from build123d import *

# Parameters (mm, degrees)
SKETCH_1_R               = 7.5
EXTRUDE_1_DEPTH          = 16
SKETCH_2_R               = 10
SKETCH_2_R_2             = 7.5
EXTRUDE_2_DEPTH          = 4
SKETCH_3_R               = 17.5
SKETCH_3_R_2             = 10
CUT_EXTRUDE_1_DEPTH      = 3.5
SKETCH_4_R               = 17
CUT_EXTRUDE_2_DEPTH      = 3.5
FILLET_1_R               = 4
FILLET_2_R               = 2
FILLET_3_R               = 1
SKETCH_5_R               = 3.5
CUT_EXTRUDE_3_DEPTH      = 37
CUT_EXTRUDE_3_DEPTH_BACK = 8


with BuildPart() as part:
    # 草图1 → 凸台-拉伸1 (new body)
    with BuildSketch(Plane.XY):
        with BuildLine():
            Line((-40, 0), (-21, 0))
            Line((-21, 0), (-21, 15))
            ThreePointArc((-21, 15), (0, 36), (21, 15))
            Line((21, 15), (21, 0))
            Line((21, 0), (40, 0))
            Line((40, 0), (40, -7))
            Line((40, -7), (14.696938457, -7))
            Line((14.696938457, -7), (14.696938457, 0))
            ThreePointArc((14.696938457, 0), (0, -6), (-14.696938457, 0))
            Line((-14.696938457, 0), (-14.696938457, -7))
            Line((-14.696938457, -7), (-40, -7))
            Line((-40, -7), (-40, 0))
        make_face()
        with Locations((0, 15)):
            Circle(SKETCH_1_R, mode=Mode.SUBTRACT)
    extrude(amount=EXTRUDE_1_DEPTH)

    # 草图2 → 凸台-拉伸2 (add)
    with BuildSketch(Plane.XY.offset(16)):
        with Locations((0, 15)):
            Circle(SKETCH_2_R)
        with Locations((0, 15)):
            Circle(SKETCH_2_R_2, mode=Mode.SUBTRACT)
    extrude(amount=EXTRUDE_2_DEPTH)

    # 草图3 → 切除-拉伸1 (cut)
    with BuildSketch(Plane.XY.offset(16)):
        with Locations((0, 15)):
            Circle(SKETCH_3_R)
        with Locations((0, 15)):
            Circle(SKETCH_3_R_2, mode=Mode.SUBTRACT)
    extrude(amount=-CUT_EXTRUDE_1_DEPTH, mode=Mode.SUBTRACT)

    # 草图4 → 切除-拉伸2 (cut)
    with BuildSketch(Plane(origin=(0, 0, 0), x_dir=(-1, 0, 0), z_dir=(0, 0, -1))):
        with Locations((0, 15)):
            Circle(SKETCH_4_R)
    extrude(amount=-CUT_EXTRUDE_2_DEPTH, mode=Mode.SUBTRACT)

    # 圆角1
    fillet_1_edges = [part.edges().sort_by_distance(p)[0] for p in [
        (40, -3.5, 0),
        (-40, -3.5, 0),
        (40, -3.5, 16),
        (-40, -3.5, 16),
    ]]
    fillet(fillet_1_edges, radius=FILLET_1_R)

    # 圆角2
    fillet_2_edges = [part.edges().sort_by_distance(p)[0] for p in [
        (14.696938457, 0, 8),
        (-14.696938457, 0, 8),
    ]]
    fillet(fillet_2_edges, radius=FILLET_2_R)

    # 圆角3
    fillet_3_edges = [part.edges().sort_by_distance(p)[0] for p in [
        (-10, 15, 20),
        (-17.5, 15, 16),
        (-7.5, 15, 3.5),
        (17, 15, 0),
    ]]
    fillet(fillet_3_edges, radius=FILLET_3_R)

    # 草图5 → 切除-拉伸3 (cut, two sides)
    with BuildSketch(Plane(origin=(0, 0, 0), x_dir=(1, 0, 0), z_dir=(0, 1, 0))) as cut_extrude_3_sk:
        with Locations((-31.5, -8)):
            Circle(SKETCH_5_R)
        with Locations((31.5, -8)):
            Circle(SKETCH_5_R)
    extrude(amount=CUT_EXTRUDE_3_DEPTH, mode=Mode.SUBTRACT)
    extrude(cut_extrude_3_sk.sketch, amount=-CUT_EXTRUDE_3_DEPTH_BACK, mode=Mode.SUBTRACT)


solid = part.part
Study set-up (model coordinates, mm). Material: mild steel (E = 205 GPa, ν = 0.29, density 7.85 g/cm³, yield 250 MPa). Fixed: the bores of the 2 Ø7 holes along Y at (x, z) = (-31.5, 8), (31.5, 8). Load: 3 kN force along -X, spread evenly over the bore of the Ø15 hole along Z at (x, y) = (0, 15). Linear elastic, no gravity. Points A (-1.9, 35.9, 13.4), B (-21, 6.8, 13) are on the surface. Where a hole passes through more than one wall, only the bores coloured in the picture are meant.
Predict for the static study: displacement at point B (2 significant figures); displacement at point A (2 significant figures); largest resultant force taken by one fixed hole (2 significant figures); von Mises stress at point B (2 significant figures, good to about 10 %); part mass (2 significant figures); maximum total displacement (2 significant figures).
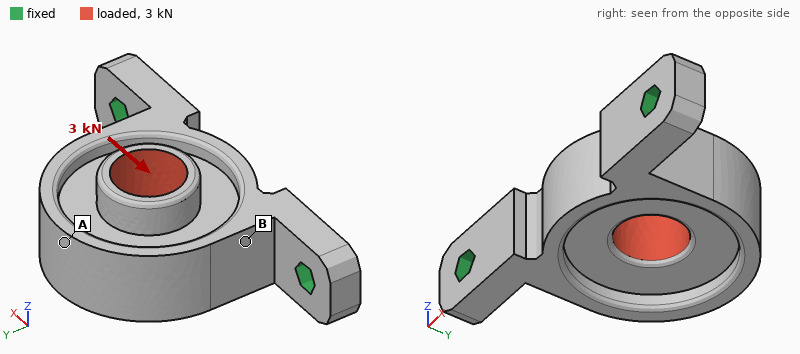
4.2 µm
9.8 µm
1.9 kN
16 MPa
170 g
11 µm
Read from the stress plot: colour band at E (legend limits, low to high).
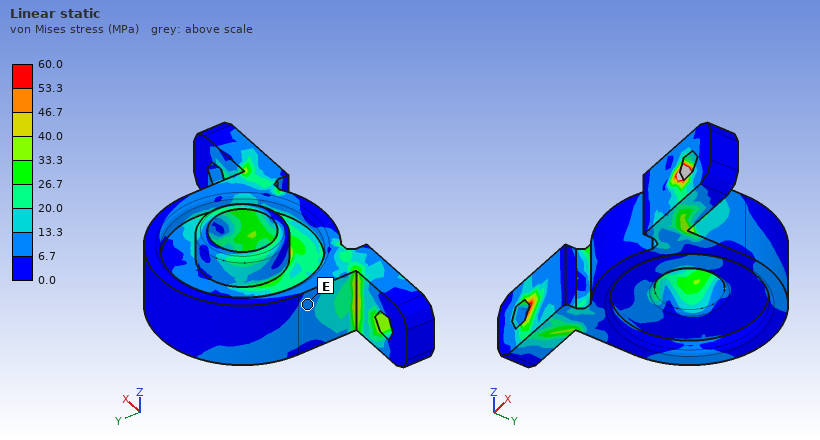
6.7 to 13.3 MPa
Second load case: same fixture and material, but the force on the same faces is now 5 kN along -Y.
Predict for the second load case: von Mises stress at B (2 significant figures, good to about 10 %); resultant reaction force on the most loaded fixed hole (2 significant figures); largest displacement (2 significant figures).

56 MPa
3.1 kN
50 µm
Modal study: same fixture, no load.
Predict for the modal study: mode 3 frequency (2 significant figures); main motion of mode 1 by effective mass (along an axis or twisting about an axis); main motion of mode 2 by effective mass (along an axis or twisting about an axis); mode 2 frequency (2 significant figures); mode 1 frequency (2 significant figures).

9700 Hz
along Z
along X
9200 Hz
2900 Hz
